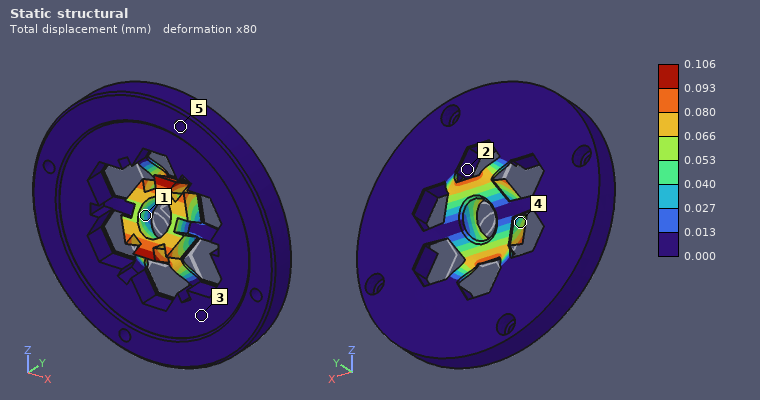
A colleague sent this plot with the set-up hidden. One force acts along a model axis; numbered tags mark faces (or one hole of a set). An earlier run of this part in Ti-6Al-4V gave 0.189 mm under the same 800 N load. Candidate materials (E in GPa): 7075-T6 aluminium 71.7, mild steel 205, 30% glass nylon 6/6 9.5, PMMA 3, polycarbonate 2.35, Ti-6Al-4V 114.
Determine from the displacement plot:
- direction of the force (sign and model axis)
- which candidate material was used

+Z
mild steel
